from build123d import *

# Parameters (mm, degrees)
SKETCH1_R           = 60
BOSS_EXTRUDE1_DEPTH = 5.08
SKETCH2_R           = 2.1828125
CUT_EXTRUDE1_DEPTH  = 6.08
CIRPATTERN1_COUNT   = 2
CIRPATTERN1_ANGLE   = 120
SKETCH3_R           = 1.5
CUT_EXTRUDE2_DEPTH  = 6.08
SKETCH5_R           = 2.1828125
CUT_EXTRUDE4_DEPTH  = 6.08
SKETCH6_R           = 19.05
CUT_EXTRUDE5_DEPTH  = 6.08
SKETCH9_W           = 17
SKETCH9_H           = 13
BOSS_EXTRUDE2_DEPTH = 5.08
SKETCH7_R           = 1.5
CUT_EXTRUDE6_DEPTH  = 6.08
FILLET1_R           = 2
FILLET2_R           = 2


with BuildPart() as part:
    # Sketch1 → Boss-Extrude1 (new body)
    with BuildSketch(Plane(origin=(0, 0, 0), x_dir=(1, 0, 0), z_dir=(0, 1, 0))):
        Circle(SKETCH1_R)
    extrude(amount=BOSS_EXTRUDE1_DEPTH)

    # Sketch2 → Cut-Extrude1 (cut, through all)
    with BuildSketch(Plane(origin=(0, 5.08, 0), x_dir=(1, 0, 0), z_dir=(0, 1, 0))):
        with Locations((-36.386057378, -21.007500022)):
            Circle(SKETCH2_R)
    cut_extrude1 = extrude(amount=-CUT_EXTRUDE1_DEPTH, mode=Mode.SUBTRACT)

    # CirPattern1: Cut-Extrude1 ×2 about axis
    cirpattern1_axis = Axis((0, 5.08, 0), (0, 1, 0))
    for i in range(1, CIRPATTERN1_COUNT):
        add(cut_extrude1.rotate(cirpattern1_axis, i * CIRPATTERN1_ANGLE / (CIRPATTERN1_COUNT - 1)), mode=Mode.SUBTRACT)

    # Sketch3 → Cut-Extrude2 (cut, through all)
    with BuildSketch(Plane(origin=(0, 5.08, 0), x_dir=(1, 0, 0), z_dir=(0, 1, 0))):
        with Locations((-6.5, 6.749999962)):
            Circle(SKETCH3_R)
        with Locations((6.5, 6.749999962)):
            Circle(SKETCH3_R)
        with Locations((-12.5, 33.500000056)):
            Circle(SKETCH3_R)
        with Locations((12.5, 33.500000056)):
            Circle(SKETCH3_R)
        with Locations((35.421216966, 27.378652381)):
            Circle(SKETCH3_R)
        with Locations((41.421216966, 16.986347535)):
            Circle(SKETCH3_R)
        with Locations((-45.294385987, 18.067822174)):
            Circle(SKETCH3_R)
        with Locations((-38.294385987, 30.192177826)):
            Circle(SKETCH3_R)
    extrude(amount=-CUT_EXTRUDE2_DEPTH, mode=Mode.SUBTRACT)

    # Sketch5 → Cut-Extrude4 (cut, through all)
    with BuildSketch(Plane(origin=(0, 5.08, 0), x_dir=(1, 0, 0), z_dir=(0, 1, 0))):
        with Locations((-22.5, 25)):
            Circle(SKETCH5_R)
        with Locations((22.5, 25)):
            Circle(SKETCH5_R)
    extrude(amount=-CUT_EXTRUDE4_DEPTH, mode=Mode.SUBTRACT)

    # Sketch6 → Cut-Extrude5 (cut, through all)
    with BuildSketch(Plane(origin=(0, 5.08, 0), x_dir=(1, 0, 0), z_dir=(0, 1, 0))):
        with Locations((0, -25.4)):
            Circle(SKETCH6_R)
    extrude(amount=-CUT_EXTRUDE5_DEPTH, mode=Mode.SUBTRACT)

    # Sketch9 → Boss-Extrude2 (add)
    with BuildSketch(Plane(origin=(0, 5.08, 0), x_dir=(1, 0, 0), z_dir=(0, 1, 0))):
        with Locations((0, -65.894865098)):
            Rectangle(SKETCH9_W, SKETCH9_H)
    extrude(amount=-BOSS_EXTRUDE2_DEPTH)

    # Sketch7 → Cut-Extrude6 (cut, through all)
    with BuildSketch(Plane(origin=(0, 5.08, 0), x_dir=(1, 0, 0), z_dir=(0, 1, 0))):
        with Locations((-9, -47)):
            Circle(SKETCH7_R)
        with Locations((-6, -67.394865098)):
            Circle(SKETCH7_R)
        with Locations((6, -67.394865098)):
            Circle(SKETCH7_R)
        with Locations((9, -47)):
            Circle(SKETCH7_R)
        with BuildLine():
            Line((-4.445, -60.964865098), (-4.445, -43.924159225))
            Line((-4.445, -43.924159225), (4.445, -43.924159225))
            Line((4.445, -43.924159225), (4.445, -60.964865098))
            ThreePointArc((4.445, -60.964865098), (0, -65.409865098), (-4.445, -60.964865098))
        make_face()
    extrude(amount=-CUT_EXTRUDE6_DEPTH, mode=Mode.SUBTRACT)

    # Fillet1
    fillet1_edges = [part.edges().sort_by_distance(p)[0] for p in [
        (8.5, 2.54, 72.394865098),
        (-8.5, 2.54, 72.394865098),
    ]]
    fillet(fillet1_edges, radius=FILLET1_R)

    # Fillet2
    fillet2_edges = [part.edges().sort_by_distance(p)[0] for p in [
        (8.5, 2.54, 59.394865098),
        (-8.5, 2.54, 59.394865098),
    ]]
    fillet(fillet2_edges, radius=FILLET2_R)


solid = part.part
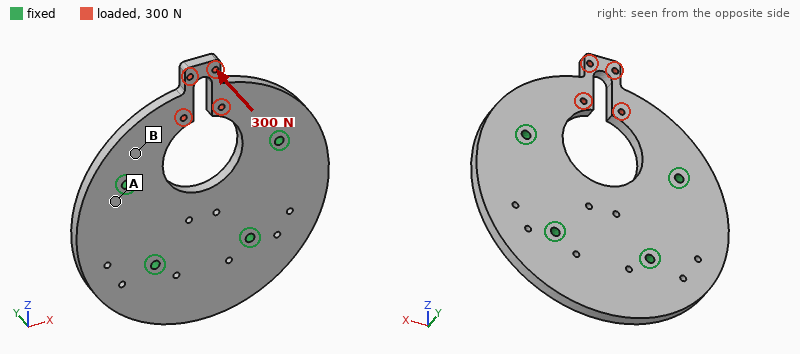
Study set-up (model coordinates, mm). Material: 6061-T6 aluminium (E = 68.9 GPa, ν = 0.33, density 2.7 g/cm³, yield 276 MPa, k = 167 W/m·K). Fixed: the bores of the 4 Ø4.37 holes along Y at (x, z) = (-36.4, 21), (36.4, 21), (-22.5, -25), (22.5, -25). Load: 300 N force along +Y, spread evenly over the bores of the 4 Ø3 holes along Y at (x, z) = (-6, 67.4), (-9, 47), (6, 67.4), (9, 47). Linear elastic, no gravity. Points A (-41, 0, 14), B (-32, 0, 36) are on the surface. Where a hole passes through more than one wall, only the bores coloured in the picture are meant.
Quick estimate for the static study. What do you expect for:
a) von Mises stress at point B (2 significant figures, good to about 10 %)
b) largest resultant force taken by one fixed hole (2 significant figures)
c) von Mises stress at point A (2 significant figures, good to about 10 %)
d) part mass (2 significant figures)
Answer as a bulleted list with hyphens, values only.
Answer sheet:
- 33 MPa
- 180 N
- 6.6 MPa
- 140 g
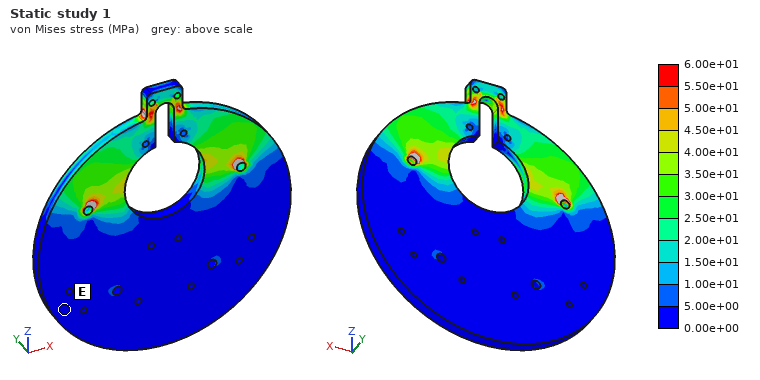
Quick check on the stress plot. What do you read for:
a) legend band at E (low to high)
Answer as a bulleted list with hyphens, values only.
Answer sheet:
- 0.00e+00 to 5.00e+00 MPa
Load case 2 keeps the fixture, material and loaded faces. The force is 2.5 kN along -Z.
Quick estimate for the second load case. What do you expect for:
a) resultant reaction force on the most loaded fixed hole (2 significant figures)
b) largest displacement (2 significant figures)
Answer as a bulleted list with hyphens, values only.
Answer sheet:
- 970 N
- 36 µm
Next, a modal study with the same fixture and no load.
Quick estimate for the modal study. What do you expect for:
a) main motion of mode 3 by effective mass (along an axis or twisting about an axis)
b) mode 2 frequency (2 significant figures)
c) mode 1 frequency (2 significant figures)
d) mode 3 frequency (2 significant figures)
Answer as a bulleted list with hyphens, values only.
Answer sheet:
- along Y
- 3700 Hz
- 1900 Hz
- 4300 Hz
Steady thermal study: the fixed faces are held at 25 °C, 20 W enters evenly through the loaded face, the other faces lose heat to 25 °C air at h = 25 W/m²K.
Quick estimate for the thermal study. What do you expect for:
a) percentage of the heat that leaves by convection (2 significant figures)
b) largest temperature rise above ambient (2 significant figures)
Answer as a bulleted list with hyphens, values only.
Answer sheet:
- 11 %
- 37 K
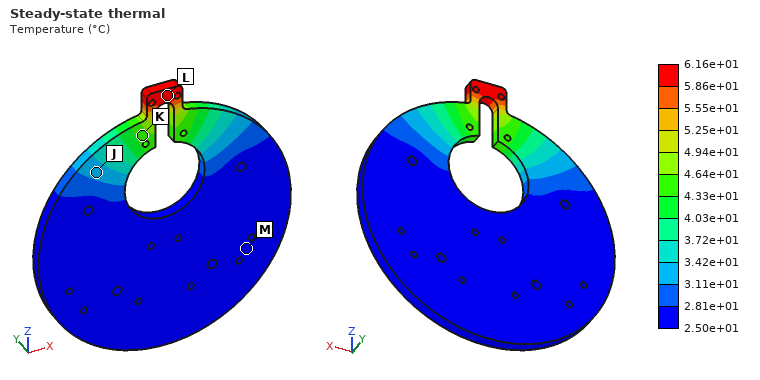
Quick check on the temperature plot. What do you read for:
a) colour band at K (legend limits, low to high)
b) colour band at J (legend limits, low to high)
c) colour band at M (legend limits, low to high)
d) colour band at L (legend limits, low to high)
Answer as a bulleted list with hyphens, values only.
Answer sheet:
- 4.33e+01 to 4.64e+01 °C
- 3.11e+01 to 3.42e+01 °C
- 2.50e+01 to 2.81e+01 °C
- 5.86e+01 to 6.16e+01 °C
